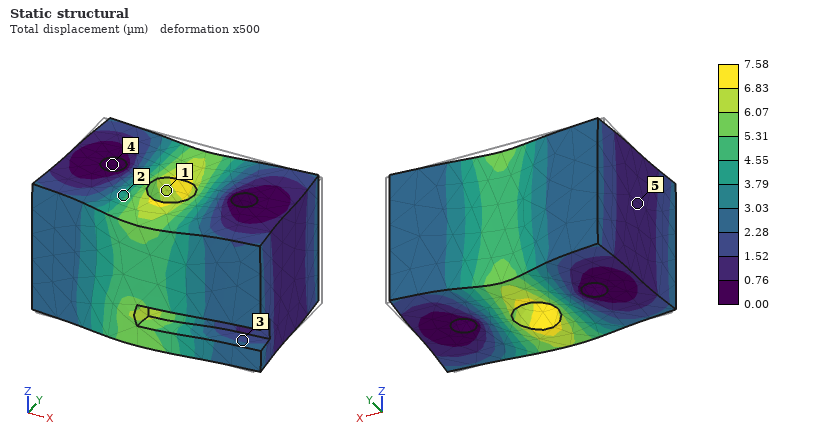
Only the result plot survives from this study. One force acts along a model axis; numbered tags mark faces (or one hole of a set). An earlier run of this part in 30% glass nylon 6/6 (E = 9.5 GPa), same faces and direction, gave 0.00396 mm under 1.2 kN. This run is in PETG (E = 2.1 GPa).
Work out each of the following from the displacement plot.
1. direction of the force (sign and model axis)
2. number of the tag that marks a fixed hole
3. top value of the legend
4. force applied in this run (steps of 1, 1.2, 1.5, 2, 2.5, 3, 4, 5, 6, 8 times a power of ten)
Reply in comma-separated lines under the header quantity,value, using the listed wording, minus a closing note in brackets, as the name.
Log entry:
quantity,value
direction of the force,-Y
number of the tag that marks a fixed hole,4
top value of the legend,7.58 µm
force applied in this run,500 N
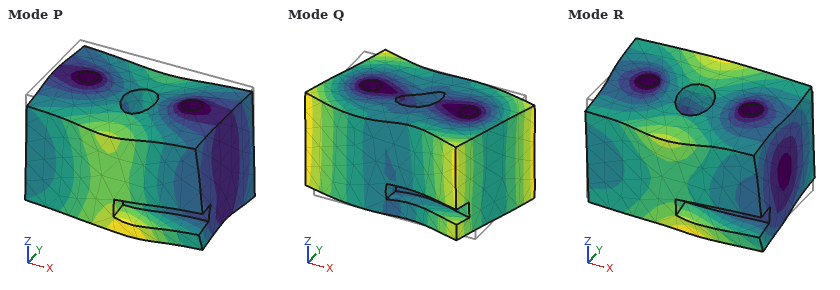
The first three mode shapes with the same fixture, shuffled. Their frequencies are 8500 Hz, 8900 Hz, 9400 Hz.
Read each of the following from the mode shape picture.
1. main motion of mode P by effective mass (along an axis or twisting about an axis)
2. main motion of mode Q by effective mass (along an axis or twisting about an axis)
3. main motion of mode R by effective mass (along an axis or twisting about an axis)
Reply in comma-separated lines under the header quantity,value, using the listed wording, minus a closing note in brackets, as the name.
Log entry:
quantity,value
main motion of mode P by effective mass,along Z
main motion of mode Q by effective mass,twisting about Z
main motion of mode R by effective mass,twisting about X
